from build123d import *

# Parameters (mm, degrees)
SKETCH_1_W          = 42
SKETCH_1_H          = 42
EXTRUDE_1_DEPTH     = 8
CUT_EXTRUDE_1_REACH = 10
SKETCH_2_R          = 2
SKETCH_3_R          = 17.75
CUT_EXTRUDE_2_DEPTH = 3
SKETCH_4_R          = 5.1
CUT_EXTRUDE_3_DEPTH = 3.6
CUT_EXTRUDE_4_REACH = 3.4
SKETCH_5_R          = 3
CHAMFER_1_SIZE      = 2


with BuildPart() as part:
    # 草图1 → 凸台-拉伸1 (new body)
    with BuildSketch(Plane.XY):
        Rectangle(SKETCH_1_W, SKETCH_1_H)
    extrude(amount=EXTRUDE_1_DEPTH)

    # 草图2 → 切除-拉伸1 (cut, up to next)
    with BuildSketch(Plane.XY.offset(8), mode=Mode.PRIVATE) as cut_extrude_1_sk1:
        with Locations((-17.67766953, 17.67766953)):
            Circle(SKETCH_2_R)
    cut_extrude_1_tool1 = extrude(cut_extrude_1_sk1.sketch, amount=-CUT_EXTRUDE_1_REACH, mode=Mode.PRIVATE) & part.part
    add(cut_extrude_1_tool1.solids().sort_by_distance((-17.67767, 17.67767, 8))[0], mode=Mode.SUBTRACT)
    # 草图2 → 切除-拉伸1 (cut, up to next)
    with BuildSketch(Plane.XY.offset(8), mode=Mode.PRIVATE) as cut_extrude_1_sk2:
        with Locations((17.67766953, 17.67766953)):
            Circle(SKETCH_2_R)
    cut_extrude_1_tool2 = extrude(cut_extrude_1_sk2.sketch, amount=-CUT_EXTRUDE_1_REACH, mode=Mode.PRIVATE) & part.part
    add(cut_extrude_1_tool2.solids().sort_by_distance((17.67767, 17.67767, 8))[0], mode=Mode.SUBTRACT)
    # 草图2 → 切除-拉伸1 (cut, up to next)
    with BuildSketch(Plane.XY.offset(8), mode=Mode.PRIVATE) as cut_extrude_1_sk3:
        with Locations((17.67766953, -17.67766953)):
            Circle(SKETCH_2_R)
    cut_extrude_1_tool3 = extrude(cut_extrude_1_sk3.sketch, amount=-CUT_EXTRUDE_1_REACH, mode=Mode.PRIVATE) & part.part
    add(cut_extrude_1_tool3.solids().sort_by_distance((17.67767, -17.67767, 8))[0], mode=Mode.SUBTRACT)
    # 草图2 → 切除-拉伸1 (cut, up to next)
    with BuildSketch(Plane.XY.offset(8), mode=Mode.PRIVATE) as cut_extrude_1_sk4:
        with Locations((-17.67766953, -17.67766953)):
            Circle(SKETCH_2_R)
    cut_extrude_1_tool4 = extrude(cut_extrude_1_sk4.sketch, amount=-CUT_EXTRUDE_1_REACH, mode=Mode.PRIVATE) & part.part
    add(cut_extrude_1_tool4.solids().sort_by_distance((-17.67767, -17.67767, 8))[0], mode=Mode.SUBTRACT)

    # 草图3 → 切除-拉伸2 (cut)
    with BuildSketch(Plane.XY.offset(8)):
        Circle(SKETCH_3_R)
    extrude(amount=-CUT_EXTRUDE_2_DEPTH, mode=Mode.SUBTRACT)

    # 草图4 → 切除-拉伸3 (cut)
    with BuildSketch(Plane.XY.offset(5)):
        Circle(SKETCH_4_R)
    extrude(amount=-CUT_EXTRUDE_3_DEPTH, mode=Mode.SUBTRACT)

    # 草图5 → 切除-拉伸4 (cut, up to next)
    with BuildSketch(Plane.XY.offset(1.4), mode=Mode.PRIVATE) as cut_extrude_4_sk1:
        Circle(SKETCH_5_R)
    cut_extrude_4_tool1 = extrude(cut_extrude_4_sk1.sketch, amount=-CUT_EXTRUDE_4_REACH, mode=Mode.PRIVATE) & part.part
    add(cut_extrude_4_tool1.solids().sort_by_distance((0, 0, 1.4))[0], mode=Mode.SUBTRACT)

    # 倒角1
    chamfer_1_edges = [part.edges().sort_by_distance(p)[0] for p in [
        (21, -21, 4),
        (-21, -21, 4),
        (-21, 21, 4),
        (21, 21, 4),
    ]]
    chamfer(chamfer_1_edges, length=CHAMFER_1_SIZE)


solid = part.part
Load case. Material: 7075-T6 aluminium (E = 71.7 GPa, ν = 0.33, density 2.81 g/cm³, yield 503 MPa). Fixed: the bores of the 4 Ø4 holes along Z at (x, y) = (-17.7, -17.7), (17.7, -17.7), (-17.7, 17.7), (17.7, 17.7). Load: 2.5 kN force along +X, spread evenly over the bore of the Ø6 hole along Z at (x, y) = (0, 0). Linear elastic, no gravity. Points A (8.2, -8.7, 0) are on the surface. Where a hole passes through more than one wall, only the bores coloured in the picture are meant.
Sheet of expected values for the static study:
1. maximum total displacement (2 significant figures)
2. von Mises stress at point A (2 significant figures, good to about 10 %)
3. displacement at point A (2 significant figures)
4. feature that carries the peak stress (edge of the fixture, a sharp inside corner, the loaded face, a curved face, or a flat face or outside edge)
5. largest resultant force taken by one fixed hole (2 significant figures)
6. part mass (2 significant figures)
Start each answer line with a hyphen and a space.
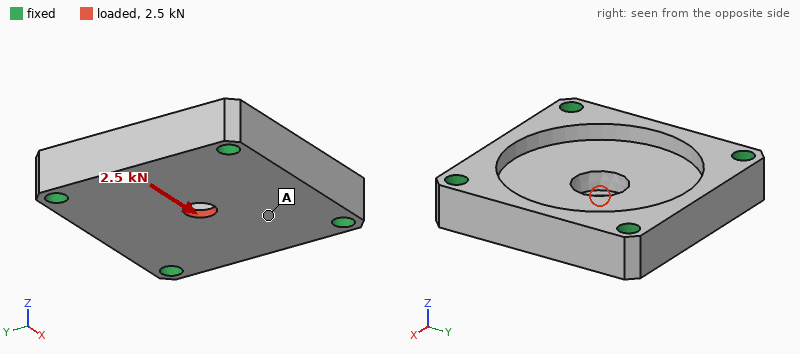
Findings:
- 11 µm
- 17 MPa
- 2.5 µm
- the loaded face
- 720 N
- 29 g
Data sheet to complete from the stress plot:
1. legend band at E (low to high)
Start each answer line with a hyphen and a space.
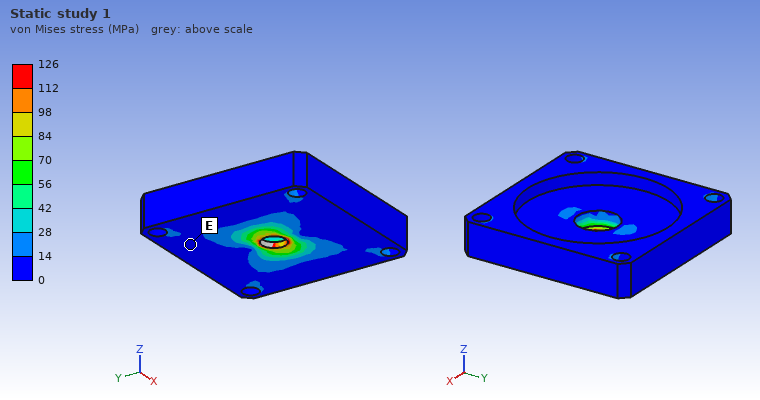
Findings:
- 0 to 14 MPa
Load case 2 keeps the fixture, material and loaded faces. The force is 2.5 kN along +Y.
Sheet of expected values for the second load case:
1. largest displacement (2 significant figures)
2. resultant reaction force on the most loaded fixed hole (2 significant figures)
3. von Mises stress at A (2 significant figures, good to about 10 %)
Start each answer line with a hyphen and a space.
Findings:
- 11 µm
- 720 N
- 18 MPa
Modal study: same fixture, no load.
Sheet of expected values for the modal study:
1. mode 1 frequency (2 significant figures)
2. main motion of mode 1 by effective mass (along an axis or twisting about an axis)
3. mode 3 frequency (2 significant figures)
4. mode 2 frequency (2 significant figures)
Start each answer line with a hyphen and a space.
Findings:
- 19 kHz
- along Z
- 28 kHz
- 28 kHz
